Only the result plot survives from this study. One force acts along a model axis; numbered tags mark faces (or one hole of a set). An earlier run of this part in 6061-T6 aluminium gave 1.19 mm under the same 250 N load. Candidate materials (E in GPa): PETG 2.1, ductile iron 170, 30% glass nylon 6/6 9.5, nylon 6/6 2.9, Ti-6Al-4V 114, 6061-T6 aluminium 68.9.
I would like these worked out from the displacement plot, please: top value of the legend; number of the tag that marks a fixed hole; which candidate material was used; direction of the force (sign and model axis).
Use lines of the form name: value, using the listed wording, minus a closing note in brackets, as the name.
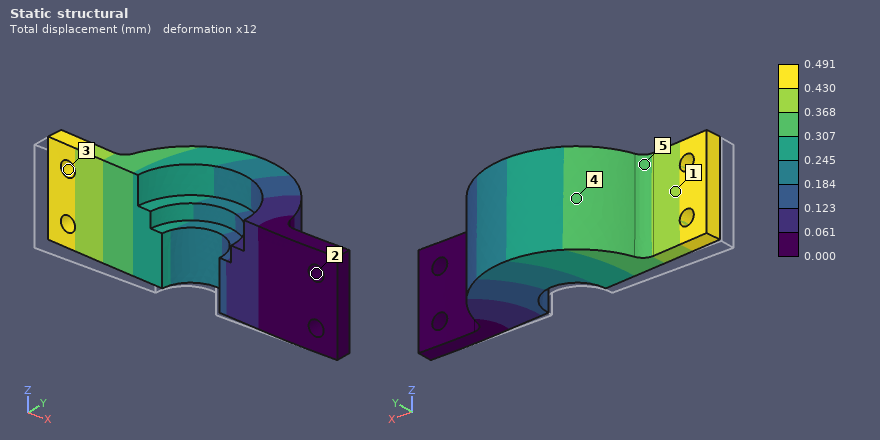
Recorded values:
top value of the legend: 0.491 mm
number of the tag that marks a fixed hole: 2
which candidate material was used: ductile iron
direction of the force: +Y
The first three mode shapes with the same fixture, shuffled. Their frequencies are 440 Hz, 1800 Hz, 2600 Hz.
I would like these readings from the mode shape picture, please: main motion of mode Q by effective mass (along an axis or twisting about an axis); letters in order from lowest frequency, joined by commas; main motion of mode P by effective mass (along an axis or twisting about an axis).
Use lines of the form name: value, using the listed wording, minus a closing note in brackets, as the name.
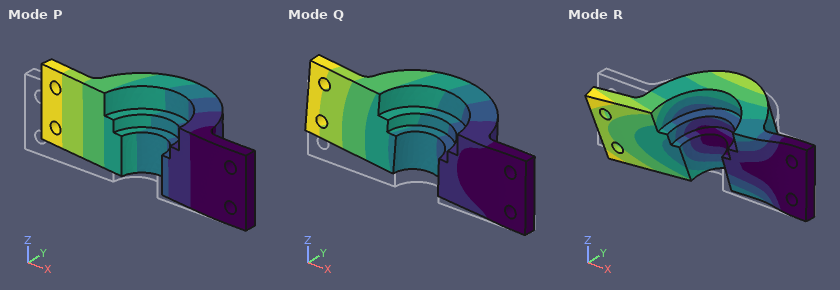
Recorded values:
main motion of mode Q by effective mass: along Z
letters in order from lowest frequency, joined by commas: P, Q, R
main motion of mode P by effective mass: along Y
